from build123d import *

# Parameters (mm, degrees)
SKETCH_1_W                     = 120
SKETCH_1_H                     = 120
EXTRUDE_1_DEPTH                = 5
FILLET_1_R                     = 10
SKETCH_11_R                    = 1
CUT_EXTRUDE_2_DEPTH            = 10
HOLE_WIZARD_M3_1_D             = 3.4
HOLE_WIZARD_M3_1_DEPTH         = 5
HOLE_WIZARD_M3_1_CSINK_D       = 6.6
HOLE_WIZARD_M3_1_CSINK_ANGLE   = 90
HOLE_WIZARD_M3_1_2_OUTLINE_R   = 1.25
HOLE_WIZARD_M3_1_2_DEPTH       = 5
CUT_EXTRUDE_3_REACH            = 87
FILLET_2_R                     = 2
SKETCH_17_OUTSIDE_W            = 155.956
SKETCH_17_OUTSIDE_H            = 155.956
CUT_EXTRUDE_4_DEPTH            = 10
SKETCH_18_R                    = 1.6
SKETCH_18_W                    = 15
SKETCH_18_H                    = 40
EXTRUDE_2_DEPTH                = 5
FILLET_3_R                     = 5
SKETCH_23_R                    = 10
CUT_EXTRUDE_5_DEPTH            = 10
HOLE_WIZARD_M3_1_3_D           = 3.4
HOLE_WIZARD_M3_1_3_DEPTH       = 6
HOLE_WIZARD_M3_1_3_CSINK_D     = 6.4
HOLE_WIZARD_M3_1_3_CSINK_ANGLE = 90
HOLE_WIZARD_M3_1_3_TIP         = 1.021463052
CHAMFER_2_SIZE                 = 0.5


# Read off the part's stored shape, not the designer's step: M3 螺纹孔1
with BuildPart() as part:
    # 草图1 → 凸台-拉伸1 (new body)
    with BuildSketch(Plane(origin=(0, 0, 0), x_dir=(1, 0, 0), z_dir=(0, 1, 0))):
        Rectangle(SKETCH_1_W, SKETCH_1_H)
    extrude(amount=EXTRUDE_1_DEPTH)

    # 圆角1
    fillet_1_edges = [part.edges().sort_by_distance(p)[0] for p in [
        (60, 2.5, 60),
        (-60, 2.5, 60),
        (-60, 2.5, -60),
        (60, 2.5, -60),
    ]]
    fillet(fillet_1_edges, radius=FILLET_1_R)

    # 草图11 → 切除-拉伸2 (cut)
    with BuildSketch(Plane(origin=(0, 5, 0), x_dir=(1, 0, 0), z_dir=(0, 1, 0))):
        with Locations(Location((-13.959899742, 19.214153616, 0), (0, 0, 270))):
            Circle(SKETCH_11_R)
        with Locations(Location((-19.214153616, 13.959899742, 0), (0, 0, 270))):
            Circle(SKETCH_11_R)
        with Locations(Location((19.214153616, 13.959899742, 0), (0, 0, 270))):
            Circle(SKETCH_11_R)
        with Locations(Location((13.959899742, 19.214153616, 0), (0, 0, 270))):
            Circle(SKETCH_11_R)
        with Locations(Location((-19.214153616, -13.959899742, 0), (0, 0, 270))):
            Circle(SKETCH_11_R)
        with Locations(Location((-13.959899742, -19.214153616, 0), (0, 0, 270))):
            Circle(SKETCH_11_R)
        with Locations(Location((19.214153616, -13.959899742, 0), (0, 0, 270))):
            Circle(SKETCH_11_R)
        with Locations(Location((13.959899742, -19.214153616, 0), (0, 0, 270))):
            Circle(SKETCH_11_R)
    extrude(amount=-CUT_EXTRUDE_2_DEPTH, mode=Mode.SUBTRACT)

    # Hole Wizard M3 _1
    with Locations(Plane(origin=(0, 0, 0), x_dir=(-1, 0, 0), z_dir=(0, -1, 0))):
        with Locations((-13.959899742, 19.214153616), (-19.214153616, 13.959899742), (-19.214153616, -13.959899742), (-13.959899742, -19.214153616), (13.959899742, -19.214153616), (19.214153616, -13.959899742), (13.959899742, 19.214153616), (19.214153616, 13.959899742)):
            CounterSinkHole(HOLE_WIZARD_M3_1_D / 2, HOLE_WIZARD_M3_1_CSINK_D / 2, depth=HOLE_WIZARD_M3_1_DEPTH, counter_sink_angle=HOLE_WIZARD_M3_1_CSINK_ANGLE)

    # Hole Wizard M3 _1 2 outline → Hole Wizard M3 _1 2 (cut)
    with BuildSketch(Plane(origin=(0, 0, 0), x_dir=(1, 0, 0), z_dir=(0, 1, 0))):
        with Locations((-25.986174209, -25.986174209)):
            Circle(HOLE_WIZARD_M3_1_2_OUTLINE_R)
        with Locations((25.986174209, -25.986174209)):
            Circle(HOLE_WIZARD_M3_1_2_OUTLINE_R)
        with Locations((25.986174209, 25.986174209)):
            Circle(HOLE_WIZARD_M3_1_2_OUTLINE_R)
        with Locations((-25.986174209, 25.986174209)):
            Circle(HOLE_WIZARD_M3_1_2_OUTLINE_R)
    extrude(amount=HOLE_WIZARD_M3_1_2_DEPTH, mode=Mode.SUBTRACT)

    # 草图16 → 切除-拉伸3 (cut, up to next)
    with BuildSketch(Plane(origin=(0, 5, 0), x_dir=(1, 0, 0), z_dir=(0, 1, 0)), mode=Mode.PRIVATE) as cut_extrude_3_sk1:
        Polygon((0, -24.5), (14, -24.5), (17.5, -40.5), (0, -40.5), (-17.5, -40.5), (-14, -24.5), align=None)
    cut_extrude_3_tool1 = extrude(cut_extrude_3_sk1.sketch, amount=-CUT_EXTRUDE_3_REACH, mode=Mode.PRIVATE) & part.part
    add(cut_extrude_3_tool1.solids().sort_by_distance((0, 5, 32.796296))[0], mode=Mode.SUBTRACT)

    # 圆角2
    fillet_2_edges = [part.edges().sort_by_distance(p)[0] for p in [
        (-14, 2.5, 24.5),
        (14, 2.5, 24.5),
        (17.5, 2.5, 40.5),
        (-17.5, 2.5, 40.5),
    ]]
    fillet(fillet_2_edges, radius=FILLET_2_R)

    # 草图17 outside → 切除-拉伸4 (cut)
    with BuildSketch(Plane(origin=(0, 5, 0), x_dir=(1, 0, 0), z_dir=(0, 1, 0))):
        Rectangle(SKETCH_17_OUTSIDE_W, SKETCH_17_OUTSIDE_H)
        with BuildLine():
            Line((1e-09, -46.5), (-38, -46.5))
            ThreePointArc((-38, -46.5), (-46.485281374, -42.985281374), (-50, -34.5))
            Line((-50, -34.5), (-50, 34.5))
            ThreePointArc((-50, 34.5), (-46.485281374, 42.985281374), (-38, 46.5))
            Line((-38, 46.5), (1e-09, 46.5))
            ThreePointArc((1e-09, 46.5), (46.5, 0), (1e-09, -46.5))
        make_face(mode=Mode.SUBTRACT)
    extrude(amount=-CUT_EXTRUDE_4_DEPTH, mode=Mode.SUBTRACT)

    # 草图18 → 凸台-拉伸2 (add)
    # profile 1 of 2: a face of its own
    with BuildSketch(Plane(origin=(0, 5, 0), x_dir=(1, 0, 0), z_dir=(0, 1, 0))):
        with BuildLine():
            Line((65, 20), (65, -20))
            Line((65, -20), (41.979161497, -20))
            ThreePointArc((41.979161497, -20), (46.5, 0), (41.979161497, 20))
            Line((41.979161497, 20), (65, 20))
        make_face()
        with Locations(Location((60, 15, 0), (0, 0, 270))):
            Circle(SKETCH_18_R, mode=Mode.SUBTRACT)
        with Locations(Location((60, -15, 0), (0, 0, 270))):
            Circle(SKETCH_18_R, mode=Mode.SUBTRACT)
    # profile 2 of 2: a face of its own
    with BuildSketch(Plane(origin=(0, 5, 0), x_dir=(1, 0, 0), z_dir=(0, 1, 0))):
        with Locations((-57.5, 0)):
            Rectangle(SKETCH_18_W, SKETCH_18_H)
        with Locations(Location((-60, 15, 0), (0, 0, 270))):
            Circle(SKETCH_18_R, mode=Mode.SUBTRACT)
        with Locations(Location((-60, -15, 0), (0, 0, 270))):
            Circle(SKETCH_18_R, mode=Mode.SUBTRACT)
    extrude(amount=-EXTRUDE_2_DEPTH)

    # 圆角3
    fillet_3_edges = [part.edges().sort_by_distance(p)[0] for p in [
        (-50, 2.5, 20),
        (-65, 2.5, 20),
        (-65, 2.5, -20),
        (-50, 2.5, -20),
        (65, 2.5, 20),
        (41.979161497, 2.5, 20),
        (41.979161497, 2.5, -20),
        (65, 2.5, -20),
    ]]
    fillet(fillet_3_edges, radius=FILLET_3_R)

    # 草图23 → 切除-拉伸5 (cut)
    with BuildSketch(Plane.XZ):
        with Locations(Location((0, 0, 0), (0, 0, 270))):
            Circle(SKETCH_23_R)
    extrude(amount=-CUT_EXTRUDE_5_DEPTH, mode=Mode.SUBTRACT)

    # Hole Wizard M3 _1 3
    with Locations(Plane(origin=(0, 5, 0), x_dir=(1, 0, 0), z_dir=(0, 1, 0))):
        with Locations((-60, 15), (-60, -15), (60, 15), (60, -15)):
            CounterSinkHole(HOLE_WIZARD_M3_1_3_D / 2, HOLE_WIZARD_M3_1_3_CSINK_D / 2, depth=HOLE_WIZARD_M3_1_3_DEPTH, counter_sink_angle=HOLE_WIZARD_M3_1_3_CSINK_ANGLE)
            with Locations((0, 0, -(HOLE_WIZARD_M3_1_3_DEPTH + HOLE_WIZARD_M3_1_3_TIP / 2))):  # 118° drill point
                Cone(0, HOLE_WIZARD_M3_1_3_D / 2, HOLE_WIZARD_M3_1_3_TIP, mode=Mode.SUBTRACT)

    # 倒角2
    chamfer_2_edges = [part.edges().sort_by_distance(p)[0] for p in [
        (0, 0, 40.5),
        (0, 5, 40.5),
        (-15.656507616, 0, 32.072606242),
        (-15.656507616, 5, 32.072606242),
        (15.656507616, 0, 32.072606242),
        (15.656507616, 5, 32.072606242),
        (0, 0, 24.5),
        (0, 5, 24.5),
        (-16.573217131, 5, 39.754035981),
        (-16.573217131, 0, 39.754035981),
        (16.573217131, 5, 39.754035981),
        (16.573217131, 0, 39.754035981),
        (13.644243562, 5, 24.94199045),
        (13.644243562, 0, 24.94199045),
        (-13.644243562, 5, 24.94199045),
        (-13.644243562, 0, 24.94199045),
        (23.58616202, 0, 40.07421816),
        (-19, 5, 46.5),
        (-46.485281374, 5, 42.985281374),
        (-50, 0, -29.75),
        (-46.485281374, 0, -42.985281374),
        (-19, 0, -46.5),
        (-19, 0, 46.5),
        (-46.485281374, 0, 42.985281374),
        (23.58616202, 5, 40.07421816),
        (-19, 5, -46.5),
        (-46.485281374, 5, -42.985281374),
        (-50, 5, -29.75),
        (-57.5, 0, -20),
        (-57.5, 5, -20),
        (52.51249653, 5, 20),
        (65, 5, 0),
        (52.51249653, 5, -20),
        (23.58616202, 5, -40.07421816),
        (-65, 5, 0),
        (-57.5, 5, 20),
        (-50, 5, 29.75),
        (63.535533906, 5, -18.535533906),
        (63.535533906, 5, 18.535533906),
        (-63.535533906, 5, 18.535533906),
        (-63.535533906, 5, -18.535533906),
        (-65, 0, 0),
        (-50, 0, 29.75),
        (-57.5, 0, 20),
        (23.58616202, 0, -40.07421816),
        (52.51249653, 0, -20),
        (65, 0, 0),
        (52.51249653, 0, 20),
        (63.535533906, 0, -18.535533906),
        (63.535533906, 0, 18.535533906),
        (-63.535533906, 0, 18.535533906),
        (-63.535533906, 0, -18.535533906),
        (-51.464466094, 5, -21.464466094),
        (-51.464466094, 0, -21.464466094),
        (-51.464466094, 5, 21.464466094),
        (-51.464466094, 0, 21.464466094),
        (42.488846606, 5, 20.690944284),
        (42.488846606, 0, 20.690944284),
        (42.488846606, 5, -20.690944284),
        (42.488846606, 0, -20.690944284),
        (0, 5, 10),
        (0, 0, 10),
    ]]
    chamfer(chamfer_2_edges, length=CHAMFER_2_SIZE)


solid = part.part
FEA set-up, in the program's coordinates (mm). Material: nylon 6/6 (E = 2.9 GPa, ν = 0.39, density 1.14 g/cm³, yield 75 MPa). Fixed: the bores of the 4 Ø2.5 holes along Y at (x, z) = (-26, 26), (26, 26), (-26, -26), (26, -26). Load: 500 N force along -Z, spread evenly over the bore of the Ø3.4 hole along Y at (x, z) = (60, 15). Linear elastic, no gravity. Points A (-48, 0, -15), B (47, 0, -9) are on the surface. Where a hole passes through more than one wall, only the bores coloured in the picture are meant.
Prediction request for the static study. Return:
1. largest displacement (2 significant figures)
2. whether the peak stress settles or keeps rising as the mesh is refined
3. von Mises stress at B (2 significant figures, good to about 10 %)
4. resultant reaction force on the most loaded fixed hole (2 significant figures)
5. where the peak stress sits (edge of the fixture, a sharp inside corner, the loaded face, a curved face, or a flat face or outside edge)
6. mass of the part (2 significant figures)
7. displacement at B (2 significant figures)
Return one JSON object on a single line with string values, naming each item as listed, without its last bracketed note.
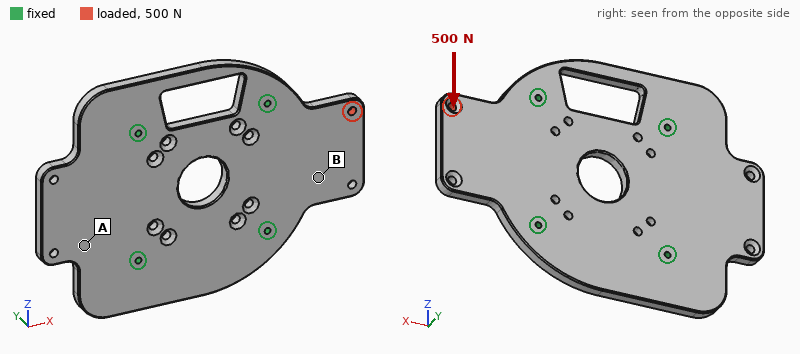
{"largest displacement": "0.24 mm", "whether the peak stress settles or keeps rising as the mesh is refined": "keeps rising", "von Mises stress at B": "5.9 MPa", "resultant reaction force on the most loaded fixed hole": "380 N", "where the peak stress sits": "a sharp inside corner", "mass of the part": "48 g", "displacement at B": "0.070 mm"}
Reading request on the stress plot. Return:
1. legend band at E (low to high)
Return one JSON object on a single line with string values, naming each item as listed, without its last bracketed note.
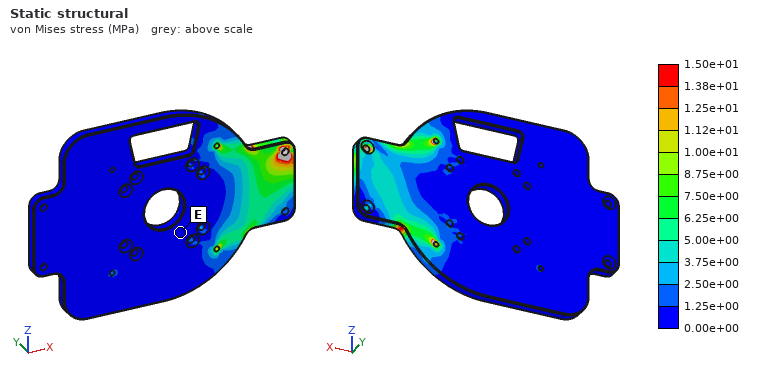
{"legend band at E": "0.00e+00 to 1.25e+00 MPa"}
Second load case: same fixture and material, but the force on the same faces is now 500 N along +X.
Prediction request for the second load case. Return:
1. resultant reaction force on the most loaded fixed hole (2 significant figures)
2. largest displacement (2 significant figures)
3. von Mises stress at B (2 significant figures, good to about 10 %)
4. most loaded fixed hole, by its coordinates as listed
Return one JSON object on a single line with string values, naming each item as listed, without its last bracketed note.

{"resultant reaction force on the most loaded fixed hole": "320 N", "largest displacement": "0.35 mm", "von Mises stress at B": "1.5 MPa", "most loaded fixed hole, by its coordinates as listed": "(26, 26)"}
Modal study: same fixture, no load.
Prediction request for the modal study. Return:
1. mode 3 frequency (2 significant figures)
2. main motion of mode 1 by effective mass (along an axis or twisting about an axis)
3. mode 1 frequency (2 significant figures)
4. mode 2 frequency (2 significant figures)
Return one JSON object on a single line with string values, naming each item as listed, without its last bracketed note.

{"mode 3 frequency": "1800 Hz", "main motion of mode 1 by effective mass": "along Y", "mode 1 frequency": "750 Hz", "mode 2 frequency": "840 Hz"}
